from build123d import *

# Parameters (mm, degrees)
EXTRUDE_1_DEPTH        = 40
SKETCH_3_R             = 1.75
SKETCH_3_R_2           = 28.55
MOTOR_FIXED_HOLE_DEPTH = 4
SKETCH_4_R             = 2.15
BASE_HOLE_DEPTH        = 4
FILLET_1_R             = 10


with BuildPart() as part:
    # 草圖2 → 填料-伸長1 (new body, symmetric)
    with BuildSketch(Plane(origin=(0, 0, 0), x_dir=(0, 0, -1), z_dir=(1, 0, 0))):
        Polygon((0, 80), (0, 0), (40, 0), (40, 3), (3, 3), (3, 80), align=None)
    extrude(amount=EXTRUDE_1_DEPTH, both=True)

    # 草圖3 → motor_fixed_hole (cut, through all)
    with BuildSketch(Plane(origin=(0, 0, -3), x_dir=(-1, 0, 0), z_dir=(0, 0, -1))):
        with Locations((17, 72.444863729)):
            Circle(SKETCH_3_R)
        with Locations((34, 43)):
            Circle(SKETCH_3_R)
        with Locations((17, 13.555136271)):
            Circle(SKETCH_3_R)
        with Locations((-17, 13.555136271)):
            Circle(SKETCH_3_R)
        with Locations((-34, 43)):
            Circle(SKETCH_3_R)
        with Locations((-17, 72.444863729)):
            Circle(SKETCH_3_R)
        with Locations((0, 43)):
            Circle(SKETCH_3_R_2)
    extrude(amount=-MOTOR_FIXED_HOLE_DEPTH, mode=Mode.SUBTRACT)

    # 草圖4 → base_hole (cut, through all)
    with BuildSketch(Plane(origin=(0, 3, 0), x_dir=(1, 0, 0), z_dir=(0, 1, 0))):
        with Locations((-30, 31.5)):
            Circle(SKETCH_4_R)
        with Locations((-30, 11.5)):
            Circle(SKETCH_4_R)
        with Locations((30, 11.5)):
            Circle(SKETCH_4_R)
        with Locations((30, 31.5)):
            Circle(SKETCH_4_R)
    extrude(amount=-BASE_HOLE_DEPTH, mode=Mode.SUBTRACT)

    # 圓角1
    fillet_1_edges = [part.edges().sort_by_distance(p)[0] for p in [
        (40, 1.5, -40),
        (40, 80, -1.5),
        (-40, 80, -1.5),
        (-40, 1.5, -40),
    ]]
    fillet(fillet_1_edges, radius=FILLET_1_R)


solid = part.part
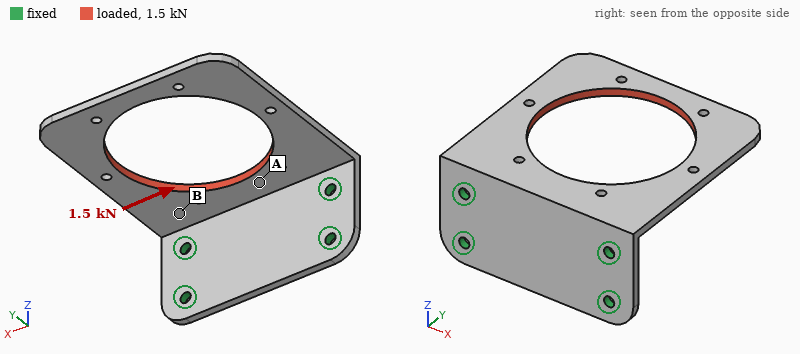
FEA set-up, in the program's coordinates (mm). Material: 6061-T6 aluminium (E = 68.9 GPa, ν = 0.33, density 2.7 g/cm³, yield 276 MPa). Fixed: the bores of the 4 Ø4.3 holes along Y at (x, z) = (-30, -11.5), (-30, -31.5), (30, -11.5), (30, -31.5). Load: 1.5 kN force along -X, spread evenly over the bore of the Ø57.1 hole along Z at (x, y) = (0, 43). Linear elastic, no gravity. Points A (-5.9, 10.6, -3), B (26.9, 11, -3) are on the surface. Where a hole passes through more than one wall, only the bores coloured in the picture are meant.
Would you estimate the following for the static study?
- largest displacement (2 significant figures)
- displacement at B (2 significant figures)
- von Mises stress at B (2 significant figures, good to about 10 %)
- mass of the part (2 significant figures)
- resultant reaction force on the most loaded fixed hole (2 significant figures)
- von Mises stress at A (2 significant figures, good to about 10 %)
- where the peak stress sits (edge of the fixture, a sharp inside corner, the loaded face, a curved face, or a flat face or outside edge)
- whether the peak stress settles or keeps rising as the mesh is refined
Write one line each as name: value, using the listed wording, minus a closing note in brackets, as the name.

largest displacement: 0.47 mm
displacement at B: 0.088 mm
von Mises stress at B: 28 MPa
mass of the part: 53 g
resultant reaction force on the most loaded fixed hole: 1.2 kN
von Mises stress at A: 70 MPa
where the peak stress sits: edge of the fixture
whether the peak stress settles or keeps rising as the mesh is refined: keeps rising
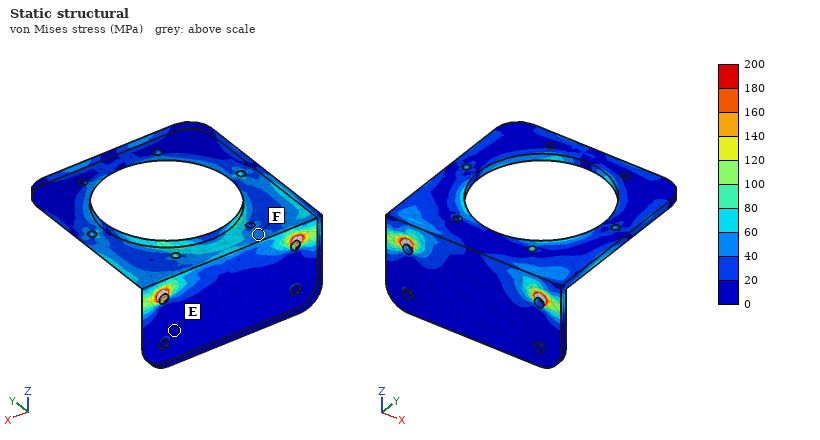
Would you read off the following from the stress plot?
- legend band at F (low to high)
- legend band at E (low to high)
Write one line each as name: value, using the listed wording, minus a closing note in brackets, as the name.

legend band at F: 40 to 60 MPa
legend band at E: 0 to 20 MPa
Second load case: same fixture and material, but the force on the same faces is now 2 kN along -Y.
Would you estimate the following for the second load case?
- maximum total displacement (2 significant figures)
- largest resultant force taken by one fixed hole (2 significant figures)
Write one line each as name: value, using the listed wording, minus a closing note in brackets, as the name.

maximum total displacement: 0.78 mm
largest resultant force taken by one fixed hole: 1.1 kN
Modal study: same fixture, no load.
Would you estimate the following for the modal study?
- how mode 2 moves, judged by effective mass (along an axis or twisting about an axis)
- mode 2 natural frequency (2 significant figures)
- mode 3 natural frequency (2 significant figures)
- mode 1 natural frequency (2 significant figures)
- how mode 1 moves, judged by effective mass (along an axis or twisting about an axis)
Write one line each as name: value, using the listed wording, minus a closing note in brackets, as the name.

how mode 2 moves, judged by effective mass: twisting about Y
mode 2 natural frequency: 720 Hz
mode 3 natural frequency: 1800 Hz
mode 1 natural frequency: 320 Hz
how mode 1 moves, judged by effective mass: along Z
